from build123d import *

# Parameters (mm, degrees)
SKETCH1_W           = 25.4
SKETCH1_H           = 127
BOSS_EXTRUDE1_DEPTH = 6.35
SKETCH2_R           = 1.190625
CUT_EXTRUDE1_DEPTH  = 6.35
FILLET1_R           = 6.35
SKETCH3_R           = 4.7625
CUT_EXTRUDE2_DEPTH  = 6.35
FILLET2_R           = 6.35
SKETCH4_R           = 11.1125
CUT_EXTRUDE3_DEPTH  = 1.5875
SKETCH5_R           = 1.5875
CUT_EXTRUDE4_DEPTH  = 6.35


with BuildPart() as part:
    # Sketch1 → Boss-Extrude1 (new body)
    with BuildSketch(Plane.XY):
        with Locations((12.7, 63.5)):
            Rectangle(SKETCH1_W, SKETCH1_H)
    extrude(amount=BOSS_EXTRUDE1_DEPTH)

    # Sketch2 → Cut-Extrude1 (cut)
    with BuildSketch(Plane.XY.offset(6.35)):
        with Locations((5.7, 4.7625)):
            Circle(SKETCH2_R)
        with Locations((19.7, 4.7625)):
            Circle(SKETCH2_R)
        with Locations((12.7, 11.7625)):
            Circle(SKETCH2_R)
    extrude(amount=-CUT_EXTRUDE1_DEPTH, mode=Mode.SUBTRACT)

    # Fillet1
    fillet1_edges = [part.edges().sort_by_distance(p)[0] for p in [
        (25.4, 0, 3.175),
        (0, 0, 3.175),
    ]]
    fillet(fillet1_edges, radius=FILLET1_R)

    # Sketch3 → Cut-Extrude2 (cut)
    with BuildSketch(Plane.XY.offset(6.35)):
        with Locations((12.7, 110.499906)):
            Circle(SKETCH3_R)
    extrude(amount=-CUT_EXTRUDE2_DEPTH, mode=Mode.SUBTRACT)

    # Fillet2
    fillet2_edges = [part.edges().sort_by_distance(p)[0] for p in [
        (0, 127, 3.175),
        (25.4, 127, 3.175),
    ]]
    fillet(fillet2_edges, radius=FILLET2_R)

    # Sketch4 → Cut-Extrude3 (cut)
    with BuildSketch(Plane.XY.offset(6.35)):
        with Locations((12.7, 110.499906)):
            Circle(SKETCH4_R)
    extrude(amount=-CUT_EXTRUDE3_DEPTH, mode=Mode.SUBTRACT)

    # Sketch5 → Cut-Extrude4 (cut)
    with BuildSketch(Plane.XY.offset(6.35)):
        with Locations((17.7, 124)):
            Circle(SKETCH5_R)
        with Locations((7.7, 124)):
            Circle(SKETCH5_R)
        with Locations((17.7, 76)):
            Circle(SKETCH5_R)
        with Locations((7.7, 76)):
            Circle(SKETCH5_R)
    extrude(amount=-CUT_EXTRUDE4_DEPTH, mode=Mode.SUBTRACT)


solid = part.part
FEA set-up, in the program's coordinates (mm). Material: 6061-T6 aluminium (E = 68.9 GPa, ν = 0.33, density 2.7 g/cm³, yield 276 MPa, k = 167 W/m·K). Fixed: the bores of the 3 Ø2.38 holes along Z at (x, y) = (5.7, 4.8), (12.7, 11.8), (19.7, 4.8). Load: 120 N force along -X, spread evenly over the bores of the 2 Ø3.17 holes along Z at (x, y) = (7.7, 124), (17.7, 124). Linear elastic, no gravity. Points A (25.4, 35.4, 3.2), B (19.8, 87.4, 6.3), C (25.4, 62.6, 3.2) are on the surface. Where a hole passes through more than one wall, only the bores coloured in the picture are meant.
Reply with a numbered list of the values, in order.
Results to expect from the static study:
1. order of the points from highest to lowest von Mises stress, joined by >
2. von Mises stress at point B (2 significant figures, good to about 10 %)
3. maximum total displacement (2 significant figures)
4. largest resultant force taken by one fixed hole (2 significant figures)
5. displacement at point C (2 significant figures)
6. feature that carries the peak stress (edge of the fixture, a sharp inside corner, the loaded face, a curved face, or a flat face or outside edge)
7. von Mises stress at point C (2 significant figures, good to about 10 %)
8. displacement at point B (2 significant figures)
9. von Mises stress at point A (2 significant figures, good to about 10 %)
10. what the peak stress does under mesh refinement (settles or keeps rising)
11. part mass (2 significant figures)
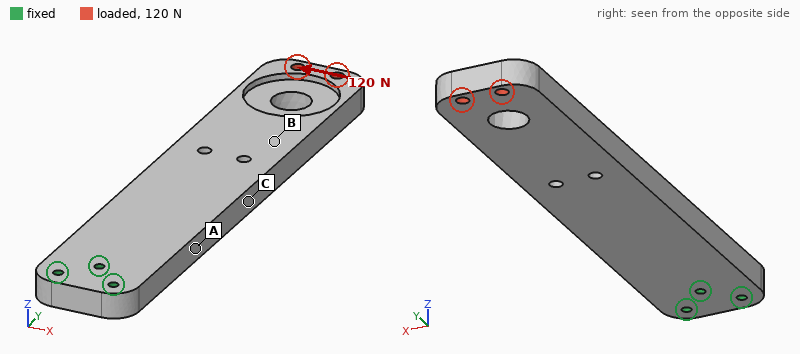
1. A > C > B
2. 3.6 MPa
3. 0.13 mm
4. 720 N
5. 0.040 mm
6. edge of the fixture
7. 11 MPa
8. 0.070 mm
9. 16 MPa
10. keeps rising
11. 51 g
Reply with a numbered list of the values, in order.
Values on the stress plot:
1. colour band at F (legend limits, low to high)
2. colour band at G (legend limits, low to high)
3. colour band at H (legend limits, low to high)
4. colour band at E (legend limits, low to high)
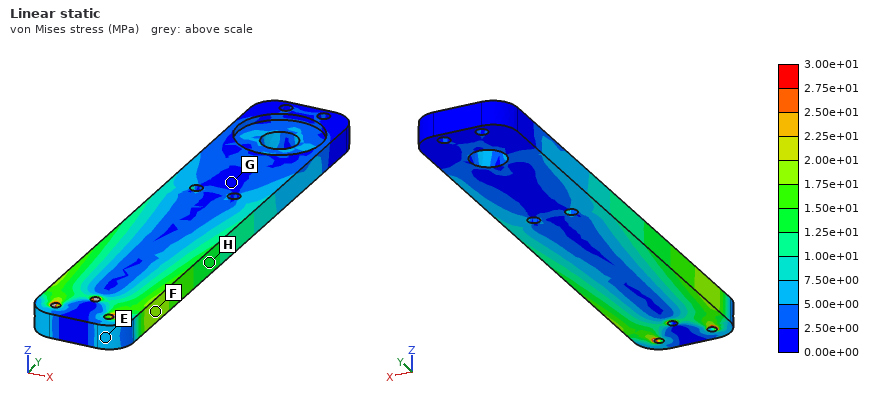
1. 1.75e+01 to 2.00e+01 MPa
2. 0.00e+00 to 2.50e+00 MPa
3. 1.25e+01 to 1.50e+01 MPa
4. 5.00e+00 to 7.50e+00 MPa
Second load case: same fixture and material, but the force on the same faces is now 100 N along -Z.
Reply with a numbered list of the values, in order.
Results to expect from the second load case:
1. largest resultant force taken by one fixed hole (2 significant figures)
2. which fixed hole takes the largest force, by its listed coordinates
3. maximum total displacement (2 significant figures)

1. 760 N
2. (12.7, 11.8)
3. 1.4 mm
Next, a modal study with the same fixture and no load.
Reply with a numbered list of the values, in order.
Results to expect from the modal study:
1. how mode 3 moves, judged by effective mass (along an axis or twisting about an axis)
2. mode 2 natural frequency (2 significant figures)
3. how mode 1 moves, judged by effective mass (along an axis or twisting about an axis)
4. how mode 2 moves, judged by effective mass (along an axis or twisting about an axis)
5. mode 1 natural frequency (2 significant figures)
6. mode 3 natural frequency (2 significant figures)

1. along Z
2. 1400 Hz
3. along Z
4. along X
5. 420 Hz
6. 2400 Hz
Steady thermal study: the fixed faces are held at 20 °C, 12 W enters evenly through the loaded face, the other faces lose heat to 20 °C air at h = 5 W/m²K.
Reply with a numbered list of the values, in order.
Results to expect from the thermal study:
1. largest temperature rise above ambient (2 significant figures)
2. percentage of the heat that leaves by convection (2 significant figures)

1. 56 K
2. 8.4 %
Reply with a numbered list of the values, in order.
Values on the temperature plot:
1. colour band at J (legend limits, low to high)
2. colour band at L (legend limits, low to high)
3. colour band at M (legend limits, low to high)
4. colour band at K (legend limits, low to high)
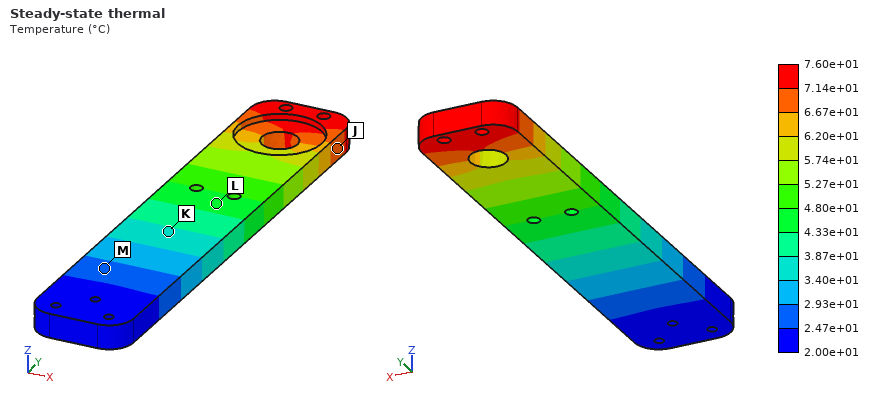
1. 6.67e+01 to 7.14e+01 °C
2. 4.33e+01 to 4.80e+01 °C
3. 2.47e+01 to 2.93e+01 °C
4. 3.40e+01 to 3.87e+01 °C
